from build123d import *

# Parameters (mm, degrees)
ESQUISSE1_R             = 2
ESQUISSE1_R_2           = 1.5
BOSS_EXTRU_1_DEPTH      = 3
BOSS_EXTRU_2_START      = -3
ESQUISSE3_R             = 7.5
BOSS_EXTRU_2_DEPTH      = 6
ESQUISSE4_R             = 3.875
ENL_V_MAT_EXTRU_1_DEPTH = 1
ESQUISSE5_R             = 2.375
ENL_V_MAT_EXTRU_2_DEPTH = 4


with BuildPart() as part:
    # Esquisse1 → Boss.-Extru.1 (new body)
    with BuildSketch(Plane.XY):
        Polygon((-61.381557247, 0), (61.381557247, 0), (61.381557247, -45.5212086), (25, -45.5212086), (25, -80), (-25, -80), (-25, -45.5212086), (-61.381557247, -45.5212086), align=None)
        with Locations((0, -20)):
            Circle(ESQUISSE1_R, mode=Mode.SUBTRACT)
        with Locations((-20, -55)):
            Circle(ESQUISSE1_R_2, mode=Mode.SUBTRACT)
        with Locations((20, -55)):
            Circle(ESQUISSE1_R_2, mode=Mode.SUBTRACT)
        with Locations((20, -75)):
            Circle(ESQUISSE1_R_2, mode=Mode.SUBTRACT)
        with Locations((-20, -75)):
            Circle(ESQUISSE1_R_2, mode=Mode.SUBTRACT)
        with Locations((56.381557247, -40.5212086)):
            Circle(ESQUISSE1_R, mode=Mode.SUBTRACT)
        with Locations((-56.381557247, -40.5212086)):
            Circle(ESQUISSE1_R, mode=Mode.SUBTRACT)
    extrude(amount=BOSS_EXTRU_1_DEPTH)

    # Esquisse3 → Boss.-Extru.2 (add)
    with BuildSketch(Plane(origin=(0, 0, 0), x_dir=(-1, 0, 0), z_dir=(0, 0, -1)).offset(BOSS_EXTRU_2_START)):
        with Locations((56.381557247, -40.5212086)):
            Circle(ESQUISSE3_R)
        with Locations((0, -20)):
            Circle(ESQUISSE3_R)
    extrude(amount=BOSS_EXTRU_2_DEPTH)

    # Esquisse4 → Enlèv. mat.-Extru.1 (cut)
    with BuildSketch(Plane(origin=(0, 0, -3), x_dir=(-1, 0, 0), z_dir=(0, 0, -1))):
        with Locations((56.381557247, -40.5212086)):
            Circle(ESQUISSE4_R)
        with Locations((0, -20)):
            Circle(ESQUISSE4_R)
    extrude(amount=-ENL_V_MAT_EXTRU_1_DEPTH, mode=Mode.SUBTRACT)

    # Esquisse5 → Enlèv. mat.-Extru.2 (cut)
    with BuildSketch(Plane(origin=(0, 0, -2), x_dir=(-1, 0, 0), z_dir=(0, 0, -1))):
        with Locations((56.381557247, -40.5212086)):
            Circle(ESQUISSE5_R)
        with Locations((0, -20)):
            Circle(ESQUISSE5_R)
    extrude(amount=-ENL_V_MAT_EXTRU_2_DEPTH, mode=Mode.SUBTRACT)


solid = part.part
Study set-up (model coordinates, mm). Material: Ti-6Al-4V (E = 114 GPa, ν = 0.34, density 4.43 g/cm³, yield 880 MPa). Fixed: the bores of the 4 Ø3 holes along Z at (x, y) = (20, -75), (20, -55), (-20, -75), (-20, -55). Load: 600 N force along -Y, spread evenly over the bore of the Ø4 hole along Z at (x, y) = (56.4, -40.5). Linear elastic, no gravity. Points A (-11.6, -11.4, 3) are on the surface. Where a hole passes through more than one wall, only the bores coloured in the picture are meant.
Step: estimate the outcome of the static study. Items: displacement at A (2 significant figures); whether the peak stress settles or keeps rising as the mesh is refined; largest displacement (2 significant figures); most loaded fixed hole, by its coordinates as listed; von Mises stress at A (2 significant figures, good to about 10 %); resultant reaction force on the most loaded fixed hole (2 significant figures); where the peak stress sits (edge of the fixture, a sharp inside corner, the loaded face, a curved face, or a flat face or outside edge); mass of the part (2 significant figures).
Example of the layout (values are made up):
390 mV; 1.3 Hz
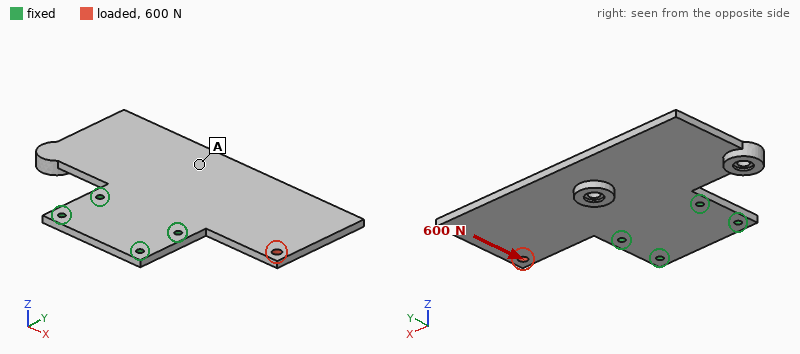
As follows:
9.9 µm; keeps rising; 32 µm; (20, -55); 6.6 MPa; 990 N; edge of the fixture; 100 g
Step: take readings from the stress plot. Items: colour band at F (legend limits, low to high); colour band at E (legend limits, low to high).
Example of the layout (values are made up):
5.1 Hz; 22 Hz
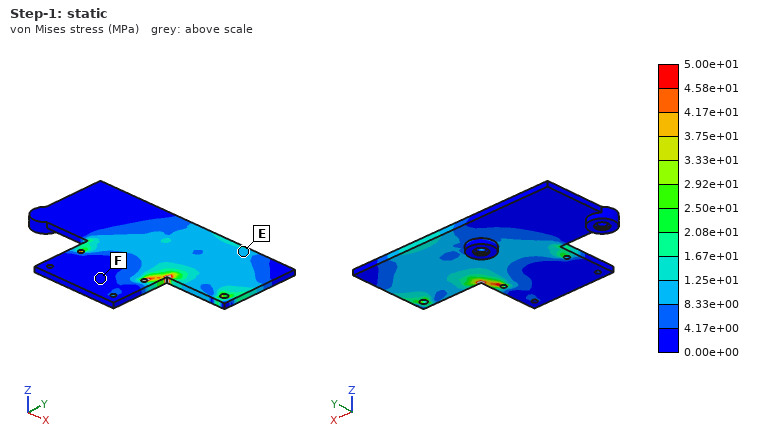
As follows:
0.00e+00 to 4.17e+00 MPa; 8.33e+00 to 1.25e+01 MPa
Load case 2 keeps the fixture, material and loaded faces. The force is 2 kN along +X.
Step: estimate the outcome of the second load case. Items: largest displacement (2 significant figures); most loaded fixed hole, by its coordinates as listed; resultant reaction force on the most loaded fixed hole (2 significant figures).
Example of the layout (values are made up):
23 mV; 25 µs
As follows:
29 µm; (20, -55); 1.3 kN
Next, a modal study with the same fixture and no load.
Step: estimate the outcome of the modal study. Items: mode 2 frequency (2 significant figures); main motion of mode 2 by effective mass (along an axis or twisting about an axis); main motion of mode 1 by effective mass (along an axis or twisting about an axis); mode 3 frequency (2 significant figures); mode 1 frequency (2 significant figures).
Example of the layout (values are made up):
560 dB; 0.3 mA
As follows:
600 Hz; twisting about Y; along Z; 1100 Hz; 510 Hz
